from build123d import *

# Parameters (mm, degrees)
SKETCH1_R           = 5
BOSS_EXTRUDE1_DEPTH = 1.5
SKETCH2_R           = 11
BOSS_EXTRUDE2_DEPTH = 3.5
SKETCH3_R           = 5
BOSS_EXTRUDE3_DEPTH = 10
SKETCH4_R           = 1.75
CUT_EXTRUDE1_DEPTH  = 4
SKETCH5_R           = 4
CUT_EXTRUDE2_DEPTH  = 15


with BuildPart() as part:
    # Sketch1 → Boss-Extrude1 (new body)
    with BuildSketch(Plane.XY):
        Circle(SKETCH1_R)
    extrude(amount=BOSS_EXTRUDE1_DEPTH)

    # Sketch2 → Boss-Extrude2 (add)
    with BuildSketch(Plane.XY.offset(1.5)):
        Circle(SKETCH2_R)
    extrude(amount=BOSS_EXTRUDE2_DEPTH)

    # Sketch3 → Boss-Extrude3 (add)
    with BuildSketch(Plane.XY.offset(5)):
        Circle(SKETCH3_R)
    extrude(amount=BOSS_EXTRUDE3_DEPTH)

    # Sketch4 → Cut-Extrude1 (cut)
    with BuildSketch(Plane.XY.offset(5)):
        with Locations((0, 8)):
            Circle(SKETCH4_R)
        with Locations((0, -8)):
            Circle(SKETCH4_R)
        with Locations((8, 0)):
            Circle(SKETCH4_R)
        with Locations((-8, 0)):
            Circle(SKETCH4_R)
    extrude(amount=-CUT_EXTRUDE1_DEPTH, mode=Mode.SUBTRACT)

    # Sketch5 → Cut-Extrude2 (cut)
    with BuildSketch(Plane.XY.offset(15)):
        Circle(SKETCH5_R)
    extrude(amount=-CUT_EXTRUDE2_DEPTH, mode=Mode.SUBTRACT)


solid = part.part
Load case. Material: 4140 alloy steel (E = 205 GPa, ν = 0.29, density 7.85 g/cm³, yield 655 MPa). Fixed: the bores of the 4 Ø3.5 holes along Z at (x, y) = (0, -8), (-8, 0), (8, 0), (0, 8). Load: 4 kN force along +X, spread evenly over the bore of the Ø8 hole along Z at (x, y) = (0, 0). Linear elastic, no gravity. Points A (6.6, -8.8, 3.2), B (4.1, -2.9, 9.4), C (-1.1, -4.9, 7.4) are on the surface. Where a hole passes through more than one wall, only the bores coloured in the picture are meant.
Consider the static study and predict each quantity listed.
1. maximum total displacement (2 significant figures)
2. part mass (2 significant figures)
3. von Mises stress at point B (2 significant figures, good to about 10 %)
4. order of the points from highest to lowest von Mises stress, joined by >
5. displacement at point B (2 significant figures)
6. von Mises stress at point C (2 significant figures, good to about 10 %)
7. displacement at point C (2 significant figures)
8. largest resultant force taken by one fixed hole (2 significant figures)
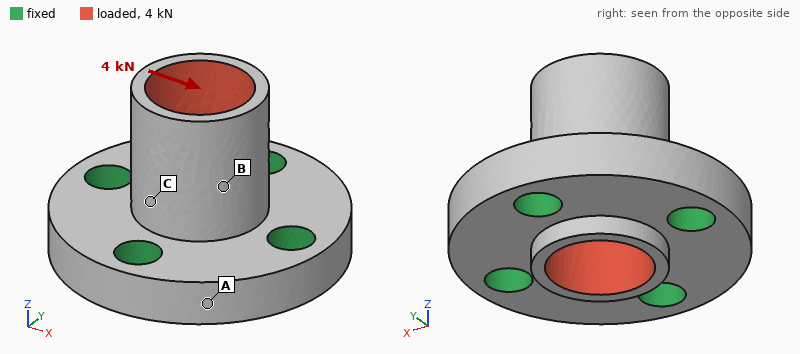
26 µm
11 g
110 MPa
C > B > A
15 µm
190 MPa
8.1 µm
1.7 kN
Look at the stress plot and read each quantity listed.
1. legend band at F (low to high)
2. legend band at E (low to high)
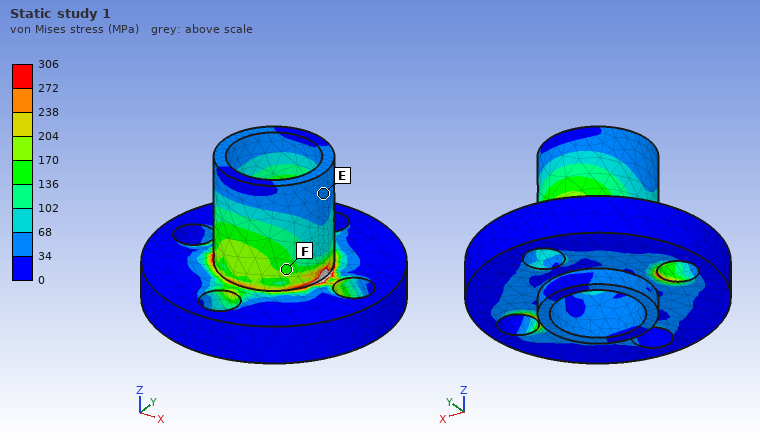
136 to 170 MPa
34 to 68 MPa
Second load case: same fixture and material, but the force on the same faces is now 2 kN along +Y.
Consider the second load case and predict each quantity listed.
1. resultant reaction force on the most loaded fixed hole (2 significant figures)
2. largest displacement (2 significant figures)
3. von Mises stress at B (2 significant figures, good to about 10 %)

840 N
13 µm
71 MPa
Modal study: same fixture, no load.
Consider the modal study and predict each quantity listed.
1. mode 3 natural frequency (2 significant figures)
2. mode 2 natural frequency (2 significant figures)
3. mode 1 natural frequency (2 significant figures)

40 kHz
40 kHz
40 kHz
